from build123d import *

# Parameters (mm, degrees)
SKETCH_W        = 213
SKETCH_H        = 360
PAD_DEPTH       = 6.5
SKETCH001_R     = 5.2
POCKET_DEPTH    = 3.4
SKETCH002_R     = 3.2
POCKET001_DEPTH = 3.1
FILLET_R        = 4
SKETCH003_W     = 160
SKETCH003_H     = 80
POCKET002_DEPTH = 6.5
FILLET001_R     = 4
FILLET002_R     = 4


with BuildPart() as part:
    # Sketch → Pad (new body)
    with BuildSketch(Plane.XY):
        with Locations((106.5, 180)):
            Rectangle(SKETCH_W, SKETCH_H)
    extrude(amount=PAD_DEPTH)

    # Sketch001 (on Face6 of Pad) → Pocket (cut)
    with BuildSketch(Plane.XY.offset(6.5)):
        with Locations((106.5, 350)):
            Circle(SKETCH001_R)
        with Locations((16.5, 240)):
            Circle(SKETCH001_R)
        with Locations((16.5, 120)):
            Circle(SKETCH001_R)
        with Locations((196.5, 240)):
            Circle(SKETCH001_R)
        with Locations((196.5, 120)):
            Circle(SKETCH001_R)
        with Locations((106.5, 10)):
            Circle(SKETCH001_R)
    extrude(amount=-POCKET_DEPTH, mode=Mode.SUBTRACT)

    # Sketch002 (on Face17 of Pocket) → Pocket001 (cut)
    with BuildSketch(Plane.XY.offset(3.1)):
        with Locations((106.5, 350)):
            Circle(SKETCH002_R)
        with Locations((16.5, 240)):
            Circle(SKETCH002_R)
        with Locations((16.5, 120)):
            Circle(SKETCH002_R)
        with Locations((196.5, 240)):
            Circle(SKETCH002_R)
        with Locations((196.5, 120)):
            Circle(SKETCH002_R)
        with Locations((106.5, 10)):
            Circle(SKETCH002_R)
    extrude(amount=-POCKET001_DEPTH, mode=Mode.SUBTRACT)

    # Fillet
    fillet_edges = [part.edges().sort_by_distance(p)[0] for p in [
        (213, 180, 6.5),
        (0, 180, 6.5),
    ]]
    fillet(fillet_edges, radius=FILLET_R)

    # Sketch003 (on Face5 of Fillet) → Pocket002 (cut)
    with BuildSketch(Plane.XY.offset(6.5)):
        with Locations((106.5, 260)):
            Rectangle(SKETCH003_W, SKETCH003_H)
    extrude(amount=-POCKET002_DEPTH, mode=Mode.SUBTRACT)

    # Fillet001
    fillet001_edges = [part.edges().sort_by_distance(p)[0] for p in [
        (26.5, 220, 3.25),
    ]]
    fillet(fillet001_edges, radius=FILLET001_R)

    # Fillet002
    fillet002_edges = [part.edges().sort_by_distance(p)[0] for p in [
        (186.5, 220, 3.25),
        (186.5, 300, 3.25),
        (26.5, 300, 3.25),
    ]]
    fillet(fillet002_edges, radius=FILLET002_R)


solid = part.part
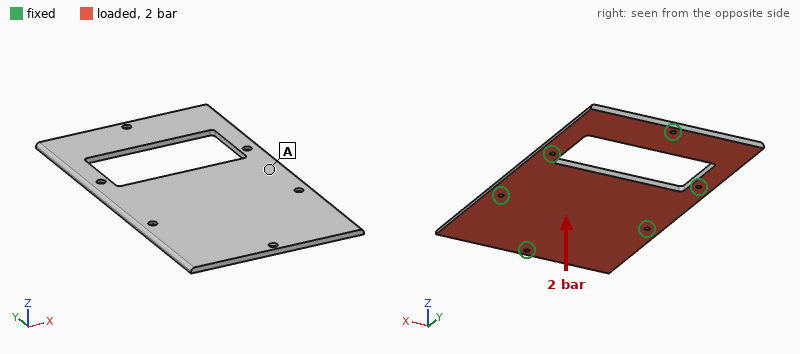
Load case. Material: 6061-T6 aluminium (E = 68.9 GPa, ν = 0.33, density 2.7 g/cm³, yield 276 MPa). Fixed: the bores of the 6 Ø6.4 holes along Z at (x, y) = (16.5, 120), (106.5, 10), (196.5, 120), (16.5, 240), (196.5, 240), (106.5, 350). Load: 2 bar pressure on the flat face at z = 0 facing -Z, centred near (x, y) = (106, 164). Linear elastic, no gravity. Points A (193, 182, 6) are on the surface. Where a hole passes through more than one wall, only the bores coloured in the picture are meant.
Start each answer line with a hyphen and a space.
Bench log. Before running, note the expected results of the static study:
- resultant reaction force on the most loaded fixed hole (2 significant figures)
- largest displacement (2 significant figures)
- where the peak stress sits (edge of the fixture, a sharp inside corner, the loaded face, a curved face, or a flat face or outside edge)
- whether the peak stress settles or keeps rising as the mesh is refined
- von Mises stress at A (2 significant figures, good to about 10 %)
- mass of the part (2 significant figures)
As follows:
- 4.1 kN
- 1.1 mm
- edge of the fixture
- keeps rising
- 27 MPa
- 1.1 kg
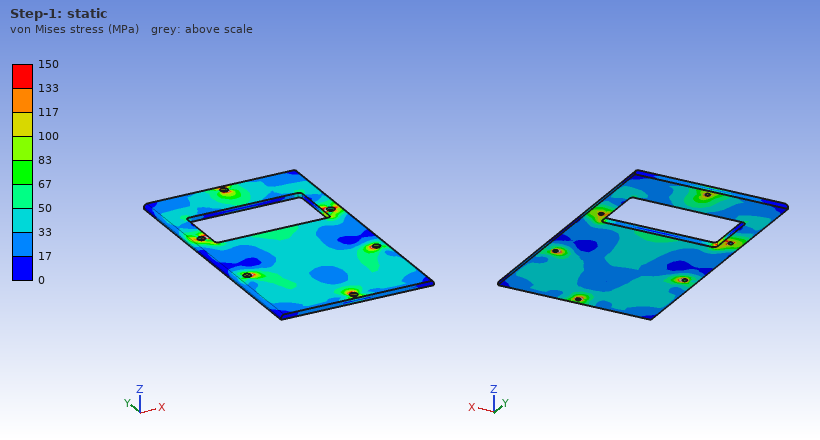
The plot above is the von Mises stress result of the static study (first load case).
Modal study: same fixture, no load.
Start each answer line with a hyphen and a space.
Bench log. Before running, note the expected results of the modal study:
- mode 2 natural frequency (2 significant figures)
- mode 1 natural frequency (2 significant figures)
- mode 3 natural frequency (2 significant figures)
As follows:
- 670 Hz
- 570 Hz
- 680 Hz
